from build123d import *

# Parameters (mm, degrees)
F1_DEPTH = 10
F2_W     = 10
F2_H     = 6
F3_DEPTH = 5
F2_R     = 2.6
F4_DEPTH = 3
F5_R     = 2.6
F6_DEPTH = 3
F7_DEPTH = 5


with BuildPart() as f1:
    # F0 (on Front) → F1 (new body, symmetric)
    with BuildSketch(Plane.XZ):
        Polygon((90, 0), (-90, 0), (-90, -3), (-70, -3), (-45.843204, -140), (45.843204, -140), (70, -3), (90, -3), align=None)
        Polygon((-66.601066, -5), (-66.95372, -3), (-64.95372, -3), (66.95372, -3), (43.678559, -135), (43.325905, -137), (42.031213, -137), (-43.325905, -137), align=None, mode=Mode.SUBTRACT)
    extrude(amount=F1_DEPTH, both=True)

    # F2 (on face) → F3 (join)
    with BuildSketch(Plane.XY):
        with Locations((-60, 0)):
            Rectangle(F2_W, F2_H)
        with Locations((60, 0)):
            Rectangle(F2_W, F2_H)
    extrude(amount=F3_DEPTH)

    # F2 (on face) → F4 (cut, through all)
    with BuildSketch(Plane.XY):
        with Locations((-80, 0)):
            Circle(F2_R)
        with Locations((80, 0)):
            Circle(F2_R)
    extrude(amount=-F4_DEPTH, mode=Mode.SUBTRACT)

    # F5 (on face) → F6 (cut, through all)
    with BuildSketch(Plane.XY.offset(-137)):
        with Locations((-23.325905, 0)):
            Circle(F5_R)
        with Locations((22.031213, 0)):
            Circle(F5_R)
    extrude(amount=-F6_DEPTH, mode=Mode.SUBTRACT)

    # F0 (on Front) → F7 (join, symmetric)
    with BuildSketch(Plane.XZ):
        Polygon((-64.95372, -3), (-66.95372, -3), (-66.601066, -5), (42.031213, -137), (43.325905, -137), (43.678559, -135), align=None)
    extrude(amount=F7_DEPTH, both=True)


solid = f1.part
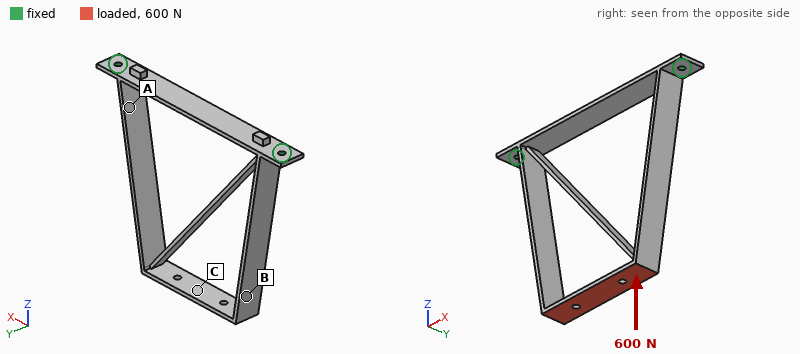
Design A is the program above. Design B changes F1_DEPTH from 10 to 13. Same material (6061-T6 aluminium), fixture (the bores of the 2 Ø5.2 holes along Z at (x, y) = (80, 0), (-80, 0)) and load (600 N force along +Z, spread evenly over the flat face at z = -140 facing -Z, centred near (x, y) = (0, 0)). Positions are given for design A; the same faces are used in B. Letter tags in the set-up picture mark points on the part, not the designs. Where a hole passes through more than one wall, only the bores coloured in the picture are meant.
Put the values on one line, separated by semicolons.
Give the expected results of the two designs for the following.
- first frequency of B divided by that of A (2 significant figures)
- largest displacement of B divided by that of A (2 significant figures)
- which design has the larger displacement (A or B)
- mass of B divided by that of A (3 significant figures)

1.0; 0.78; A; 1.26
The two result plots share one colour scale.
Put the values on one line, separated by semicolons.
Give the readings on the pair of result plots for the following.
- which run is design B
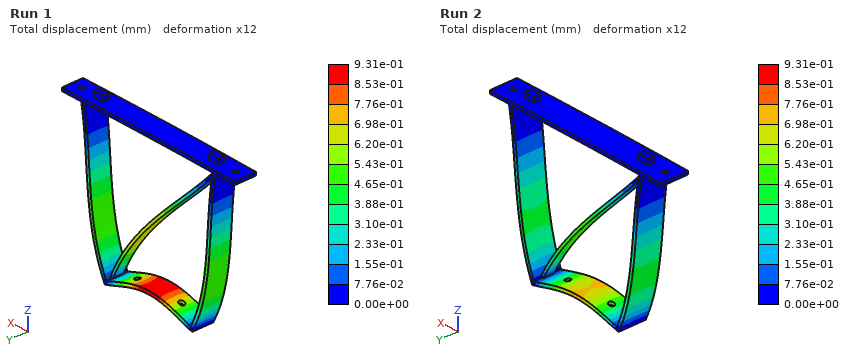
Run 2
